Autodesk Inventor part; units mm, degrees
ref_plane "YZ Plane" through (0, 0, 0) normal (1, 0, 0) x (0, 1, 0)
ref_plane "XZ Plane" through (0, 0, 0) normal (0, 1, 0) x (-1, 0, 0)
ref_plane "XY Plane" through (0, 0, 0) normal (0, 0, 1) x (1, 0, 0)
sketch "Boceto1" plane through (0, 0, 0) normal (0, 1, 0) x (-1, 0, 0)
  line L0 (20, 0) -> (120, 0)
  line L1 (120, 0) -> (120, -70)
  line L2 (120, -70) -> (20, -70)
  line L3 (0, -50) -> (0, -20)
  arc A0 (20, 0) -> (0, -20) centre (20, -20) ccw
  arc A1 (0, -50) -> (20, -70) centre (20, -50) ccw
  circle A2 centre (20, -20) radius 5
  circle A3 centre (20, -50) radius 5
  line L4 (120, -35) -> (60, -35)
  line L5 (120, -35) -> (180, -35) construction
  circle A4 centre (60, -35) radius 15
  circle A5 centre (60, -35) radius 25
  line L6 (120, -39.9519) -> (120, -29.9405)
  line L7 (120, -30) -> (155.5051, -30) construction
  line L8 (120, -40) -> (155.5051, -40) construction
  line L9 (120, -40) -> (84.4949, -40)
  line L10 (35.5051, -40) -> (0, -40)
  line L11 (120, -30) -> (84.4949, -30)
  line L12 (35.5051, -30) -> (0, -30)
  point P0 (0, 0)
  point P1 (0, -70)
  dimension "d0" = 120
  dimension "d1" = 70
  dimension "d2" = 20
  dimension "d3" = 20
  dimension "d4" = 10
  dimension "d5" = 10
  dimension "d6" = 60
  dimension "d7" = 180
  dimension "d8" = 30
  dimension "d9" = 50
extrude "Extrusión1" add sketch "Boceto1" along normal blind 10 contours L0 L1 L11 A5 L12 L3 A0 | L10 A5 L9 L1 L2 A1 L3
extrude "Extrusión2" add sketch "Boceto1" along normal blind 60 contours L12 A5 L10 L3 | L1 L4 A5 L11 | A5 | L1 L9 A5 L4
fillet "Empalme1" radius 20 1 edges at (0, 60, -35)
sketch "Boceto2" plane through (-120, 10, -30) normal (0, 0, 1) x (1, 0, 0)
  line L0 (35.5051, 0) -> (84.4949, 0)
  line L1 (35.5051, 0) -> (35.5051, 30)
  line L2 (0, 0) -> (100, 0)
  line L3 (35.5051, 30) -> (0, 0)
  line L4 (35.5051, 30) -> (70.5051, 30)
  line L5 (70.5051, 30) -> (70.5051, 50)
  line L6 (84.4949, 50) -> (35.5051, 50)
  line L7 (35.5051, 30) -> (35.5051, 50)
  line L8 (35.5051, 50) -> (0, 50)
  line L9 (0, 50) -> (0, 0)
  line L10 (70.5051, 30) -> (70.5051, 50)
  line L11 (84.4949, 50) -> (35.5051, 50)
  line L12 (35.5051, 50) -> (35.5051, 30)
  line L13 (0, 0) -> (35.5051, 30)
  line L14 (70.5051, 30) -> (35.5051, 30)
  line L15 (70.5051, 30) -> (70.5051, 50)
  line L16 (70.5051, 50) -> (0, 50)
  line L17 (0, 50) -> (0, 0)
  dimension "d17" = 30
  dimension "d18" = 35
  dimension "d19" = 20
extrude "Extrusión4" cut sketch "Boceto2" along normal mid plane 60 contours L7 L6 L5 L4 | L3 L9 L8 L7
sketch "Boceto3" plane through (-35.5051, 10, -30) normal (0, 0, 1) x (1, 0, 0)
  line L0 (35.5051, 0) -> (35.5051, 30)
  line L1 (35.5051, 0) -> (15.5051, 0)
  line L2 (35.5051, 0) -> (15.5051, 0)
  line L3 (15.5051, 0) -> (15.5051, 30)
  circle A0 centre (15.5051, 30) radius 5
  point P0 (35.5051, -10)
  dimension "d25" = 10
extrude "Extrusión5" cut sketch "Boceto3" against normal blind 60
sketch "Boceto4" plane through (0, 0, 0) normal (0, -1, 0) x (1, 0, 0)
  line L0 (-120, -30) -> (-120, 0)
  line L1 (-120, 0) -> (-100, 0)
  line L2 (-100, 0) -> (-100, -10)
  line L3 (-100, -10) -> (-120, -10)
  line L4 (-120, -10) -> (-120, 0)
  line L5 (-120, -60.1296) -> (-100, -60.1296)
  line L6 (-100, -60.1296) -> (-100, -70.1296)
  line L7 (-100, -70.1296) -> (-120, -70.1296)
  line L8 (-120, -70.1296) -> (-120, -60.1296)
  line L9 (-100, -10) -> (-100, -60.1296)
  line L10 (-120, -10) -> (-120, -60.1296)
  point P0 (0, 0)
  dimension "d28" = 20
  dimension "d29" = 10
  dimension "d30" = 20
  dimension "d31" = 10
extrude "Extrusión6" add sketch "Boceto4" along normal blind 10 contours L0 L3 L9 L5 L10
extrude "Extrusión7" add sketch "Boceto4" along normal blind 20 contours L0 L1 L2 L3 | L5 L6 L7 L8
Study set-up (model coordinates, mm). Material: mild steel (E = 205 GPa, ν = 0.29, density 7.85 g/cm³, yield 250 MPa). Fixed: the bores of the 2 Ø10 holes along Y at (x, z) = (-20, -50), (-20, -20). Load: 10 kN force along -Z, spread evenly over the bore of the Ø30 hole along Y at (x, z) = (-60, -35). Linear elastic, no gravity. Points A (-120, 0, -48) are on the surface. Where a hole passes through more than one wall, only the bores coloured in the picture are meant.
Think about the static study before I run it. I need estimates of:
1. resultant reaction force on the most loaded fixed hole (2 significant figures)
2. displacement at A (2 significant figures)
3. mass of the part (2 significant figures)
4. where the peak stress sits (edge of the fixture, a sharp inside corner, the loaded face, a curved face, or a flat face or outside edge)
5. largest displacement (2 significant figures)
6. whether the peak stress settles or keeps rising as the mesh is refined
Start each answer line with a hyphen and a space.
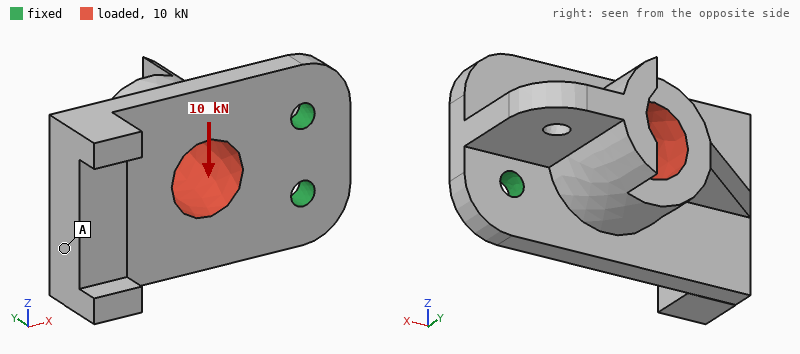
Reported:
- 12 kN
- 28 µm
- 1.2 kg
- edge of the fixture
- 56 µm
- keeps rising
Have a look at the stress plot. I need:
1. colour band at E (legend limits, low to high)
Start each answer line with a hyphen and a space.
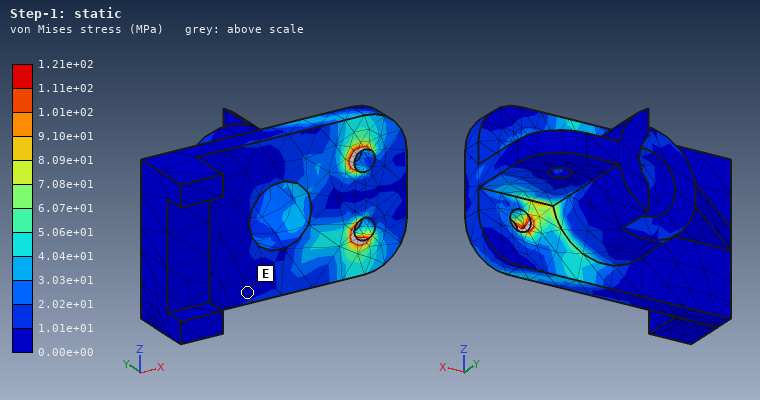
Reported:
- 0.00e+00 to 1.01e+01 MPa
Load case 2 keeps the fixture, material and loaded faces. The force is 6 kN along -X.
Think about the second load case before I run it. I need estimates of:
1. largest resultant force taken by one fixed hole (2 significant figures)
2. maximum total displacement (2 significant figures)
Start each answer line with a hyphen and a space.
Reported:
- 3.0 kN
- 59 µm
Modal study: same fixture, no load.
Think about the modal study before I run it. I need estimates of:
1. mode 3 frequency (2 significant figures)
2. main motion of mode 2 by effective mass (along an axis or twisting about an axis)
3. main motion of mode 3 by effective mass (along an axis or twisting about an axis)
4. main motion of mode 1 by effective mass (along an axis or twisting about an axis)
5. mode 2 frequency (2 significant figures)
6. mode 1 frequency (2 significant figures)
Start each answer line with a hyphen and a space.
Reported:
- 2600 Hz
- along Z
- along Z
- along Y
- 2300 Hz
- 1100 Hz
